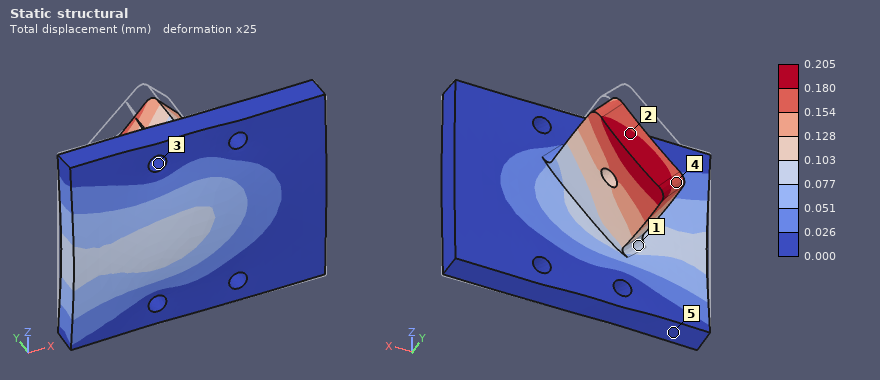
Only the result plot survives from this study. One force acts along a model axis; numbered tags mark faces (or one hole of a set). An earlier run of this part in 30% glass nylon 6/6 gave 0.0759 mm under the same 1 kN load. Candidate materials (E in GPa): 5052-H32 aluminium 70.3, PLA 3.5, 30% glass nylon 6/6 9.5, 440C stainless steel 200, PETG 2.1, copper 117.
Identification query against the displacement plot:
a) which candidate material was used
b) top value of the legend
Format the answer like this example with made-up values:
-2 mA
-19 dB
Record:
PLA
0.205 mm
